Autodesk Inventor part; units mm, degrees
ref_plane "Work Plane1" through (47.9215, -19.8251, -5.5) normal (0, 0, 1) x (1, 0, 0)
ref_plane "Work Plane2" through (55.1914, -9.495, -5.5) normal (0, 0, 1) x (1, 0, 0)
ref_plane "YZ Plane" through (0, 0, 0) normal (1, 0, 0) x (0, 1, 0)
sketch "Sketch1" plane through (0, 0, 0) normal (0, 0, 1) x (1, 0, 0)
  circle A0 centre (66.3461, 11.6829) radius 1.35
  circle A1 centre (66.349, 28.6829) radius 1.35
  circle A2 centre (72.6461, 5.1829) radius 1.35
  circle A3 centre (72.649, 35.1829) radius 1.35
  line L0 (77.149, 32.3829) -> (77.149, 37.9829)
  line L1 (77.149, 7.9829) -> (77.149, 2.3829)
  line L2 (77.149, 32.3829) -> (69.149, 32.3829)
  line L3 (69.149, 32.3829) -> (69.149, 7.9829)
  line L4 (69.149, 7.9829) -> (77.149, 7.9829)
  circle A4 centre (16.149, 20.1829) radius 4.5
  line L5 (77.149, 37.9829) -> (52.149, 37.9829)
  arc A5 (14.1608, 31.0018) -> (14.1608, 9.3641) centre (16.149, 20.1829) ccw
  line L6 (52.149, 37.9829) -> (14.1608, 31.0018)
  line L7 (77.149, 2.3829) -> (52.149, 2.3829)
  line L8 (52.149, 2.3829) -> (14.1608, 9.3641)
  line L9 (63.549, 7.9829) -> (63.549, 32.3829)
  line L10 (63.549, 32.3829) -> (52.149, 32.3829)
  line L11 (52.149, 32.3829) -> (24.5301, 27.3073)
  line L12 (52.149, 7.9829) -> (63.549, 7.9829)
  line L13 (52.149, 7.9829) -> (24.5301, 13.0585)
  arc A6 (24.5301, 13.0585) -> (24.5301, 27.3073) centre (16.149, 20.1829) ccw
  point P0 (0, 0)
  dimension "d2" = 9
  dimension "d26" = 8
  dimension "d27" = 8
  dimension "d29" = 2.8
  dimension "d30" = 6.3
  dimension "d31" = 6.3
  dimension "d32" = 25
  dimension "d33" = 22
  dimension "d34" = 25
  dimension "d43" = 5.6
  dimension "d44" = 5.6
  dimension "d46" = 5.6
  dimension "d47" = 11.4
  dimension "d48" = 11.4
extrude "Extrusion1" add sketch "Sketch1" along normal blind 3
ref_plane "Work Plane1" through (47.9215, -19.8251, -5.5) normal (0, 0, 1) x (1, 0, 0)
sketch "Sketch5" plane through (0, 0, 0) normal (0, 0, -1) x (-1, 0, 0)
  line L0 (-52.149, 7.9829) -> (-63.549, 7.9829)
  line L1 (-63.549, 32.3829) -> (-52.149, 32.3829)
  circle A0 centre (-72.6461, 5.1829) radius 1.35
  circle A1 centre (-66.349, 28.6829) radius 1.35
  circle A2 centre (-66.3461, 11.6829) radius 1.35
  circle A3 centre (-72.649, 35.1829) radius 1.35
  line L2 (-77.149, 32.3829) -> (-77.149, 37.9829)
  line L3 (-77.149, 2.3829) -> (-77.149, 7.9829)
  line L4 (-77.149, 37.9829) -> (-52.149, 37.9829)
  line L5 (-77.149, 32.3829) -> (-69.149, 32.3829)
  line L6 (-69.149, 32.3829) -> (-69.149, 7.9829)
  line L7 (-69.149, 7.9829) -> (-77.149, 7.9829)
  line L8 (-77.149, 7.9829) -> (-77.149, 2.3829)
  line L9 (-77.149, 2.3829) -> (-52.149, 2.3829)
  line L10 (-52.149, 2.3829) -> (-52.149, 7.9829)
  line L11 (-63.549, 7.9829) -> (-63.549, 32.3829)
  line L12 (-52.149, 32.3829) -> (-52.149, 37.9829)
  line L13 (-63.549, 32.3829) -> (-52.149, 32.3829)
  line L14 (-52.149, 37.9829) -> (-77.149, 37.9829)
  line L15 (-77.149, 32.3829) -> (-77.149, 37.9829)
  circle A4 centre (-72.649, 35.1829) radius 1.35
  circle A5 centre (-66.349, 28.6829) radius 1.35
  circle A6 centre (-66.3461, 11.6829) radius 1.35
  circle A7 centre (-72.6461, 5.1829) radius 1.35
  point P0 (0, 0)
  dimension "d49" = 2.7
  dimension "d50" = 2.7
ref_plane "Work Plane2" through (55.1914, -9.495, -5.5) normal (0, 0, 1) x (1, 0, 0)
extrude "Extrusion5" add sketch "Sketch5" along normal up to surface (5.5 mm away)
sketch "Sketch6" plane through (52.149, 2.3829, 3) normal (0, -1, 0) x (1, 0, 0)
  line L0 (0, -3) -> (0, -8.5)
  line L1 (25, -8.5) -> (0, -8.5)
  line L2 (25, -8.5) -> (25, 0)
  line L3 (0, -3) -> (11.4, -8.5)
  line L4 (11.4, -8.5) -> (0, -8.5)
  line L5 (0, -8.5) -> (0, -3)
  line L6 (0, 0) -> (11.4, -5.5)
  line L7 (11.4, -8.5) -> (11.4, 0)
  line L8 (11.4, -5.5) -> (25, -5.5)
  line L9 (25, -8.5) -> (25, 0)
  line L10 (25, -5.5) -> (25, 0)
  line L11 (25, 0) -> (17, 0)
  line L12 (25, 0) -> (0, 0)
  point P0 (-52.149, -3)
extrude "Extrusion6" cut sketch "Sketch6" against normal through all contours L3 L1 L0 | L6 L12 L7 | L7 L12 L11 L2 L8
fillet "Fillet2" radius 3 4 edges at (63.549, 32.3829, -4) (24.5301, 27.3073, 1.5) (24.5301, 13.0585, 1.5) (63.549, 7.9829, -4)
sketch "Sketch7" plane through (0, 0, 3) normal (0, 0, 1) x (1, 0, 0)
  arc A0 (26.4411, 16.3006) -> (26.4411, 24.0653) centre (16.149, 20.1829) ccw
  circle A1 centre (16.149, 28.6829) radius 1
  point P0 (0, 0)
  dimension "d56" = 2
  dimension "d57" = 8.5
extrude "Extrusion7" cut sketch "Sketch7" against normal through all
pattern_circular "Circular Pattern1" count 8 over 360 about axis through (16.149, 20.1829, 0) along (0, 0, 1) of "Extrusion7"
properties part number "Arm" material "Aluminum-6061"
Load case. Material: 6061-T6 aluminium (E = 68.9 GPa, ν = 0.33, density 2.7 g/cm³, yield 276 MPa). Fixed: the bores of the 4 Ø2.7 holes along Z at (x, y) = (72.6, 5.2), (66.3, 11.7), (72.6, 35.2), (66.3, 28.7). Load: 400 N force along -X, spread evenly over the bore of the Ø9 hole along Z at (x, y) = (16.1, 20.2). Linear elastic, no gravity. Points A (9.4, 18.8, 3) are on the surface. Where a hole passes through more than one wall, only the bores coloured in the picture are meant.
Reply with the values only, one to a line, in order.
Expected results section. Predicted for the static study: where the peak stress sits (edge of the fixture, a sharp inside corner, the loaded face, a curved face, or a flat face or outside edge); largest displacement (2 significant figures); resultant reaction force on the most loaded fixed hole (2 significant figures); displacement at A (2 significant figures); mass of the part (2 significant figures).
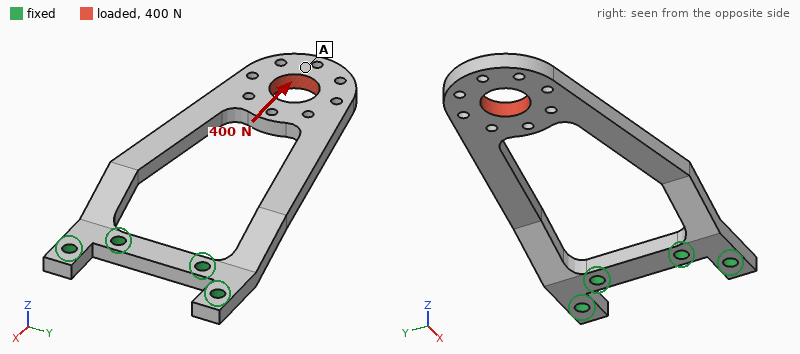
a curved face
0.81 mm
220 N
0.75 mm
8.4 g
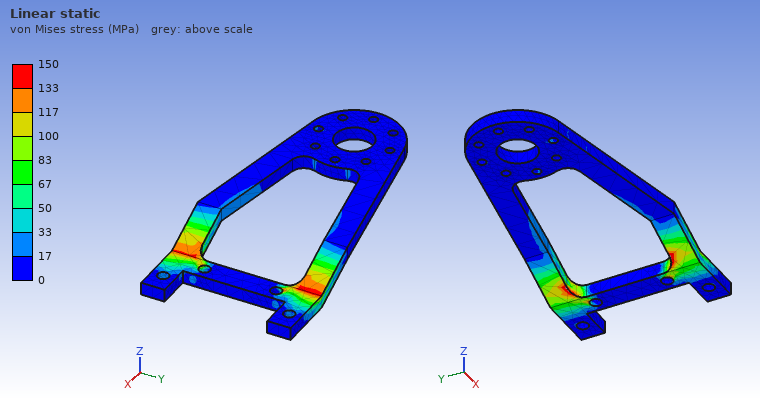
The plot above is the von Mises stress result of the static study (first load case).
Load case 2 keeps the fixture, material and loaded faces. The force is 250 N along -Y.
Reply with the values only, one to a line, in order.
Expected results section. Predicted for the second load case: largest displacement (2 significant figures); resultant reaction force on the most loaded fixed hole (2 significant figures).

0.32 mm
490 N
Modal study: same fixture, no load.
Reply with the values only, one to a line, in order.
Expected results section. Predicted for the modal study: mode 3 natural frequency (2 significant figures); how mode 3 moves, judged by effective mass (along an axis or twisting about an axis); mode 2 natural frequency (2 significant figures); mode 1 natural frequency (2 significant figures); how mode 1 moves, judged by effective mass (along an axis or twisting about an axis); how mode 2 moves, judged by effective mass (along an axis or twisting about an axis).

2900 Hz
along Y
2100 Hz
510 Hz
along Z
along Y
